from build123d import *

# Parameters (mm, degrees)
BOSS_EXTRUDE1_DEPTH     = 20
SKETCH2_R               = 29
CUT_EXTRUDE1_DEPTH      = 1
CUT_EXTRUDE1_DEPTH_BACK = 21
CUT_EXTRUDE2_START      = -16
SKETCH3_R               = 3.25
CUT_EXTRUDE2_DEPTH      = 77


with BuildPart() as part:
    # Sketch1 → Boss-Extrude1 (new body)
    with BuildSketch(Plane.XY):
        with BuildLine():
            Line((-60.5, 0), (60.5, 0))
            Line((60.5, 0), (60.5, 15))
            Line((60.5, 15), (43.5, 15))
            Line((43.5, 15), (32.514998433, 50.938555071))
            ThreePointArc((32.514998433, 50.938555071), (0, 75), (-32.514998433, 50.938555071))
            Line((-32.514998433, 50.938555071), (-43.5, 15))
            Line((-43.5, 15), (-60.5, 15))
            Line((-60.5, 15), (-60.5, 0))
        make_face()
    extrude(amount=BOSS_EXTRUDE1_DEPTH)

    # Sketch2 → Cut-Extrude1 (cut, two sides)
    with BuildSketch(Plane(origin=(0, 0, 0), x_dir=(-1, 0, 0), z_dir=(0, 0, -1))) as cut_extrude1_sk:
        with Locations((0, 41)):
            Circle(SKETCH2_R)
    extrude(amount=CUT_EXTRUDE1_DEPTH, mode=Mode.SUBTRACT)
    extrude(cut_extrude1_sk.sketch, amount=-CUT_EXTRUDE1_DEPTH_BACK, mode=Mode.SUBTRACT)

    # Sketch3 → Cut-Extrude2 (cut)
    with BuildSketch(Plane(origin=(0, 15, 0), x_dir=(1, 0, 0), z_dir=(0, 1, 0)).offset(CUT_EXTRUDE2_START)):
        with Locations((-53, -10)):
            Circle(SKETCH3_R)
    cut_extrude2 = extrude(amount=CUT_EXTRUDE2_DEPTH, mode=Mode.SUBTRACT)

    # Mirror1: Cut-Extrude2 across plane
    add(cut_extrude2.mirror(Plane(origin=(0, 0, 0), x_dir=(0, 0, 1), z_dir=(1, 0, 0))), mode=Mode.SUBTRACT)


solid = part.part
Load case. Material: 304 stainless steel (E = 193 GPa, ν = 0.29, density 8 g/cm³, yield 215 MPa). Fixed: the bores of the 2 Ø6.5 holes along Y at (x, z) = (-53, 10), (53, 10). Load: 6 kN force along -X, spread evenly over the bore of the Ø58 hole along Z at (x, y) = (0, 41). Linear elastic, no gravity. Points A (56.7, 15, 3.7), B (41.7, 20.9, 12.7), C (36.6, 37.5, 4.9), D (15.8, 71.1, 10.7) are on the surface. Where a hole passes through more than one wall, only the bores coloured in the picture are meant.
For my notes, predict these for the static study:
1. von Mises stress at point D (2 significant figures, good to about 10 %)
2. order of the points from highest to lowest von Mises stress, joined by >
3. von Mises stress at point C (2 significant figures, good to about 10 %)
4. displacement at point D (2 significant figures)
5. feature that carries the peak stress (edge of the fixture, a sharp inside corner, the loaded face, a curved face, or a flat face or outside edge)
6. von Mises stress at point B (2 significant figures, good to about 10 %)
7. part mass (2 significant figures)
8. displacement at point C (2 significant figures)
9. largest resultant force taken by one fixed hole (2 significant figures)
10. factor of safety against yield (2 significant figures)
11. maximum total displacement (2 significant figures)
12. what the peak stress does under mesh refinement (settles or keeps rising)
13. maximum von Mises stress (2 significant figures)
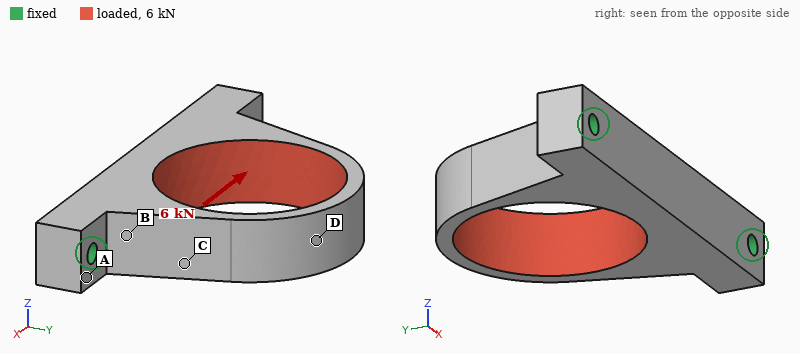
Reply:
66 MPa
C > D > B > A
89 MPa
79 µm
the loaded face
43 MPa
480 g
16 µm
3.6 kN
2.0
82 µm
settles
110 MPa
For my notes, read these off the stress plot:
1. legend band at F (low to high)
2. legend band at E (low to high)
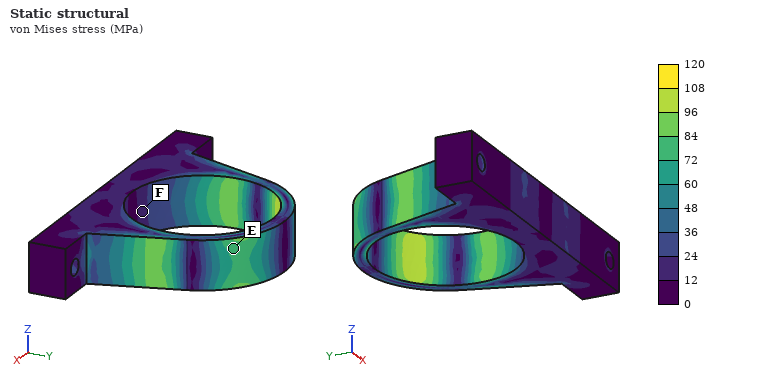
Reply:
12 to 24 MPa
72 to 84 MPa
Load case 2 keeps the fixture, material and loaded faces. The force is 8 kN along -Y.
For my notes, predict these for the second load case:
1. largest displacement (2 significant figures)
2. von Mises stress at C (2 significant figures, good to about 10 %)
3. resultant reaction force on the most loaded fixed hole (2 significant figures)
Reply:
19 µm
44 MPa
4.0 kN
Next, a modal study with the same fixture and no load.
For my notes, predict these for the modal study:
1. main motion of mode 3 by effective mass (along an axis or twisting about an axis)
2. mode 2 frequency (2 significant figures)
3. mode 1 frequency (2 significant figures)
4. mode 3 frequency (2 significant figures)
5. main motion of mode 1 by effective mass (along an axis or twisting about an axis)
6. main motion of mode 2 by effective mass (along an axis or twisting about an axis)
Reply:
along Y
3700 Hz
2500 Hz
4800 Hz
along Z
along X
